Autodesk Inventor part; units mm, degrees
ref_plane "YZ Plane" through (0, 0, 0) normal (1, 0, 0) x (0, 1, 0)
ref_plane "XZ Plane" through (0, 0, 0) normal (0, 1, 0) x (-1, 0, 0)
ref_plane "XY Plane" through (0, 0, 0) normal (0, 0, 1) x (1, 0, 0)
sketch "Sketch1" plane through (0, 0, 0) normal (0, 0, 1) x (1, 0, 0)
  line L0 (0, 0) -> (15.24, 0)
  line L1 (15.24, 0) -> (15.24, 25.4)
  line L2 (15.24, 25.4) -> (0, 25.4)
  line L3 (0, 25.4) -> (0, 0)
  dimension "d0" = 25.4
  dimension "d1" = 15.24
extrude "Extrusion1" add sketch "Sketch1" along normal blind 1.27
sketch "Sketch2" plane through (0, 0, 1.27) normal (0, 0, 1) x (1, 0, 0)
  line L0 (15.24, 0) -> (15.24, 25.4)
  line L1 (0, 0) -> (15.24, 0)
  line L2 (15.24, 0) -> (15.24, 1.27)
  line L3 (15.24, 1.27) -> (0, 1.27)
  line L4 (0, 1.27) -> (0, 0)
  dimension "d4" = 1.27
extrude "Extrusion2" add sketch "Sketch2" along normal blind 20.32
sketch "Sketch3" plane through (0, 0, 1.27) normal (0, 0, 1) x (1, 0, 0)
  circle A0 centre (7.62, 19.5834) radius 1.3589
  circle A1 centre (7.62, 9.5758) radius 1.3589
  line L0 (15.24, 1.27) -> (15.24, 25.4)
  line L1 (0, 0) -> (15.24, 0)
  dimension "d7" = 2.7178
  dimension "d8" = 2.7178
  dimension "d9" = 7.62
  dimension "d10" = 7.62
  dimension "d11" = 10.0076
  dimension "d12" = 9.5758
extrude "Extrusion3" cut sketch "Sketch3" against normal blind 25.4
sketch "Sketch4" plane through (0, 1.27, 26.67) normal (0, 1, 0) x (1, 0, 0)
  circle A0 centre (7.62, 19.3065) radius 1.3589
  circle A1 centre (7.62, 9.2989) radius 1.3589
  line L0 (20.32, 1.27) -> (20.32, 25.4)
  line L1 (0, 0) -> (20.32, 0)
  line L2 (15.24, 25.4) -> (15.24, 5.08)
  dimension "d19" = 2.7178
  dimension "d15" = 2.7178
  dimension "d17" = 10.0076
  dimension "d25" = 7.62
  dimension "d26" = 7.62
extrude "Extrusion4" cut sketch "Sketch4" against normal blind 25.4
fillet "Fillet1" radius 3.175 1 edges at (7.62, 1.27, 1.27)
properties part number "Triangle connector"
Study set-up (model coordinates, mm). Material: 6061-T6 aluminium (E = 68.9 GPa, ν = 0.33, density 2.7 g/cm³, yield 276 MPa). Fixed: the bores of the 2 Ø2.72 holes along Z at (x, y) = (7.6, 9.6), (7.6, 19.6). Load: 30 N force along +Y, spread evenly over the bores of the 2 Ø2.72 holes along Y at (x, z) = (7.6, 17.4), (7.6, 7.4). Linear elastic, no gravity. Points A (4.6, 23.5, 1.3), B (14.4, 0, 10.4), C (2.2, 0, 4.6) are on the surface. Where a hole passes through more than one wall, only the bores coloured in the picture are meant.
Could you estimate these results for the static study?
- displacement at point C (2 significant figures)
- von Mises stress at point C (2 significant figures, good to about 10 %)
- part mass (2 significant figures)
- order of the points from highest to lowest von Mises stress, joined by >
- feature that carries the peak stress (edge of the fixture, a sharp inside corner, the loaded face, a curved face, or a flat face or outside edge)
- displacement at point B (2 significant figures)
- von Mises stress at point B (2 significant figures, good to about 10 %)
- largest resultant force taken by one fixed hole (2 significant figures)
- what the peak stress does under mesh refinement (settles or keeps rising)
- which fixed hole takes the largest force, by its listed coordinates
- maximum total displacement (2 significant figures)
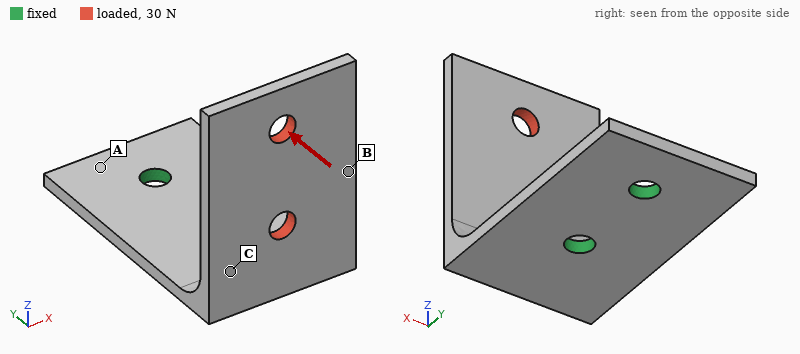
0.092 mm
53 MPa
2.4 g
C > B > A
edge of the fixture
0.17 mm
29 MPa
27 N
keeps rising
(7.6, 9.6)
0.41 mm
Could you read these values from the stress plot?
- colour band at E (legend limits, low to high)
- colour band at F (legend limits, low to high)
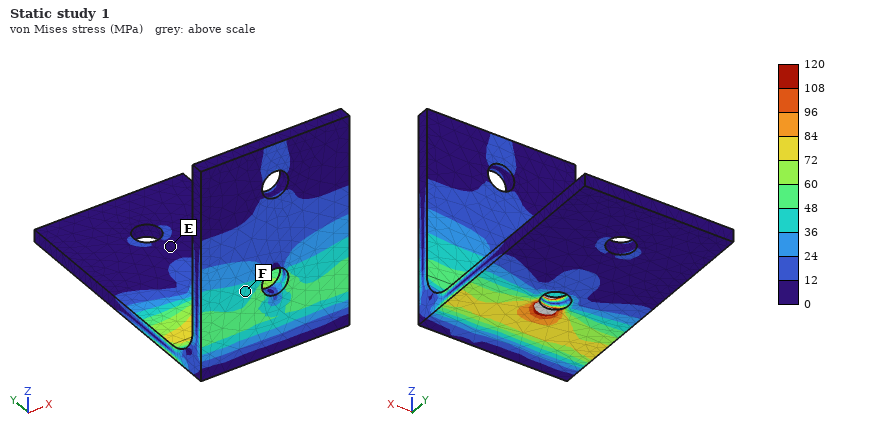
0 to 12 MPa
36 to 48 MPa
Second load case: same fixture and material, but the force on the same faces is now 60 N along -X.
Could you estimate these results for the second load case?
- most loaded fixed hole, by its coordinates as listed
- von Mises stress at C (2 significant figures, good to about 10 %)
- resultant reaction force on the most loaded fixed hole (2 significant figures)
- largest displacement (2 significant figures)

(7.6, 9.6)
23 MPa
96 N
0.29 mm
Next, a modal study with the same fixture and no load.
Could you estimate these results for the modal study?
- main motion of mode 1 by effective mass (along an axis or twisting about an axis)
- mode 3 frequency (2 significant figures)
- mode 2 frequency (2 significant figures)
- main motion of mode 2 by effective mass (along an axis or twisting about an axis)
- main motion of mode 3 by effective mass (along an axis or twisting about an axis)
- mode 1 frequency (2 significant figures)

along Y
6100 Hz
2700 Hz
along X
along Z
1700 Hz
